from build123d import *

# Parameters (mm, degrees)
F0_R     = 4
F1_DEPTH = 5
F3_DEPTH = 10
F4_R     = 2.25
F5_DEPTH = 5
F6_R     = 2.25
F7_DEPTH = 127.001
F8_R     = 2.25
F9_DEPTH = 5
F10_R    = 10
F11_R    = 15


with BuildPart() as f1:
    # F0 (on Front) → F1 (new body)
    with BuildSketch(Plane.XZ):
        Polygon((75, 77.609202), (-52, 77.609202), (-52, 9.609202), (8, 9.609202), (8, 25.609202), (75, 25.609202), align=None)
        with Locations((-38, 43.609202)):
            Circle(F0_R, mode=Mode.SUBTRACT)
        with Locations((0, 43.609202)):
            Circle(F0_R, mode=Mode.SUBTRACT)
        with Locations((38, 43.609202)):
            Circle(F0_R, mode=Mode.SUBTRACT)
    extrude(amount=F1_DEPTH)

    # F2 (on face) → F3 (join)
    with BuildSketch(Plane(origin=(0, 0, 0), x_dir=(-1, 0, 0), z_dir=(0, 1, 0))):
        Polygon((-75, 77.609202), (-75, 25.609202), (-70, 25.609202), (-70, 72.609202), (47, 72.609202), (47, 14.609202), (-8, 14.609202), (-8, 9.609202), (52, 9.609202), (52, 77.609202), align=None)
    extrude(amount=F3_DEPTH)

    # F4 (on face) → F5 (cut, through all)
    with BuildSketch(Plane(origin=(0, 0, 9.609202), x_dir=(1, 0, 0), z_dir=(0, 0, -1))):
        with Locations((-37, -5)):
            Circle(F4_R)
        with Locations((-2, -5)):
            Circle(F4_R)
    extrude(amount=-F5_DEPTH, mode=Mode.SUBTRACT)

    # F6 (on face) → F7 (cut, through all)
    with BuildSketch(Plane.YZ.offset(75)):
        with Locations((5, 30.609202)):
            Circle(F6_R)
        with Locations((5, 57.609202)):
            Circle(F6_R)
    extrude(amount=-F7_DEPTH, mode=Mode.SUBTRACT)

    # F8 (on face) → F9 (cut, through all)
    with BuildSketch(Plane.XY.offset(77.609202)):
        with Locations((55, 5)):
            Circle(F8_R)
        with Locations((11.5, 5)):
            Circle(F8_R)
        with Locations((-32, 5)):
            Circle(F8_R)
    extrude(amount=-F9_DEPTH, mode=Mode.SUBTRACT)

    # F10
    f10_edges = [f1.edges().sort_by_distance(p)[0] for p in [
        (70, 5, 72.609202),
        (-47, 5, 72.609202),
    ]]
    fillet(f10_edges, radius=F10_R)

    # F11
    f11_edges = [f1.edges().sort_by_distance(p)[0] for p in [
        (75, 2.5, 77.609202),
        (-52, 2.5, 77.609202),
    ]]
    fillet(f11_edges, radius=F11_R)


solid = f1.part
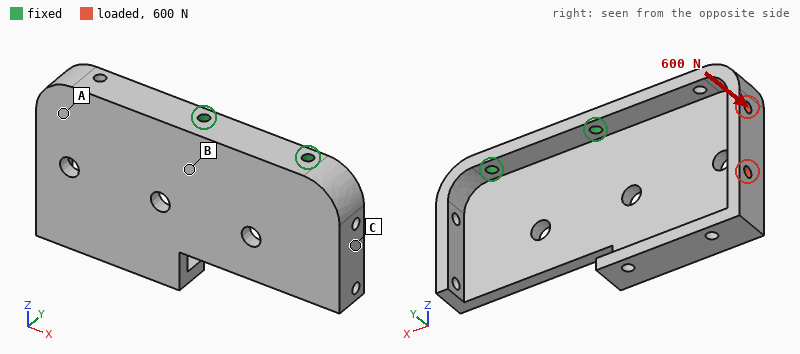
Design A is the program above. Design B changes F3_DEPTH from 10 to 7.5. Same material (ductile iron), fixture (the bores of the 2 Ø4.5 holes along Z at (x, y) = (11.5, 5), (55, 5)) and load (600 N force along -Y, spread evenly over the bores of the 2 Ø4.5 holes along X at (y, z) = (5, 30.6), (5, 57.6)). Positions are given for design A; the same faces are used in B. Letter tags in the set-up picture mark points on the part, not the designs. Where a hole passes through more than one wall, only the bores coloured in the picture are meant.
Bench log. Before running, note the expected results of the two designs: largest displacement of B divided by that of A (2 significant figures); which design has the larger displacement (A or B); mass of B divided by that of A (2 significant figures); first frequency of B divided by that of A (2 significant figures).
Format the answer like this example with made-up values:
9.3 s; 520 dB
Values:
1.2; B; 0.93; 0.97
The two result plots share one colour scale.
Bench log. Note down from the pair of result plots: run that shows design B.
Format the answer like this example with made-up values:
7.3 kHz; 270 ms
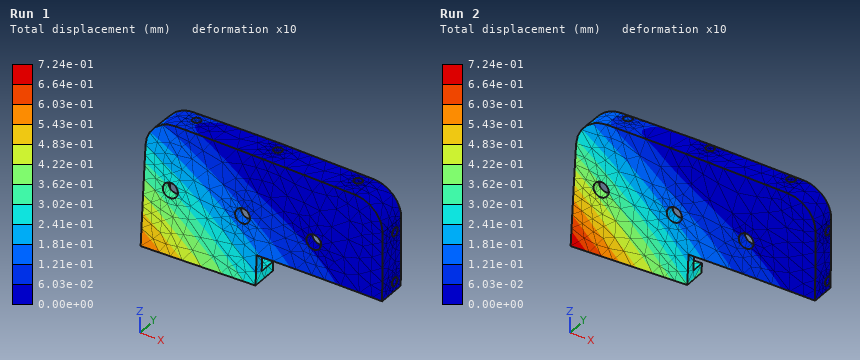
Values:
Run 2
